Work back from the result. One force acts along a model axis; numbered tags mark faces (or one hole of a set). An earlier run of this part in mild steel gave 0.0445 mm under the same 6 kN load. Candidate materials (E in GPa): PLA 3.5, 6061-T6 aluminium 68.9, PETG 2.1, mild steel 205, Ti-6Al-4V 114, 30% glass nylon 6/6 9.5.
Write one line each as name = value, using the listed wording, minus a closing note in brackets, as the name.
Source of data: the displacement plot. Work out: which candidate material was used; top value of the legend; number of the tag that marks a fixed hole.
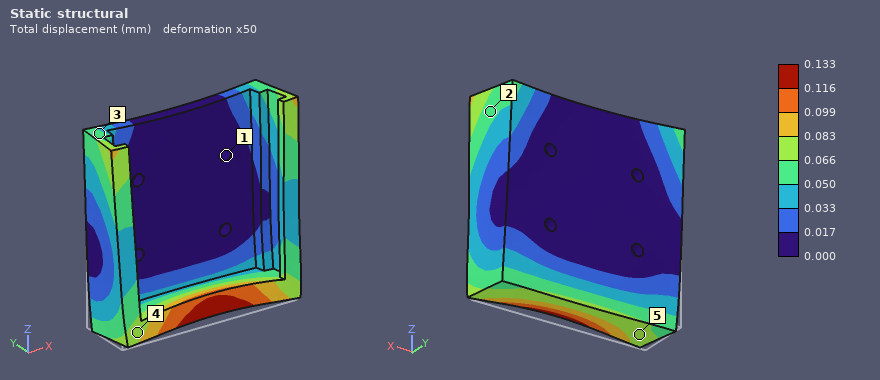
which candidate material was used = 6061-T6 aluminium
top value of the legend = 0.133 mm
number of the tag that marks a fixed hole = 1
